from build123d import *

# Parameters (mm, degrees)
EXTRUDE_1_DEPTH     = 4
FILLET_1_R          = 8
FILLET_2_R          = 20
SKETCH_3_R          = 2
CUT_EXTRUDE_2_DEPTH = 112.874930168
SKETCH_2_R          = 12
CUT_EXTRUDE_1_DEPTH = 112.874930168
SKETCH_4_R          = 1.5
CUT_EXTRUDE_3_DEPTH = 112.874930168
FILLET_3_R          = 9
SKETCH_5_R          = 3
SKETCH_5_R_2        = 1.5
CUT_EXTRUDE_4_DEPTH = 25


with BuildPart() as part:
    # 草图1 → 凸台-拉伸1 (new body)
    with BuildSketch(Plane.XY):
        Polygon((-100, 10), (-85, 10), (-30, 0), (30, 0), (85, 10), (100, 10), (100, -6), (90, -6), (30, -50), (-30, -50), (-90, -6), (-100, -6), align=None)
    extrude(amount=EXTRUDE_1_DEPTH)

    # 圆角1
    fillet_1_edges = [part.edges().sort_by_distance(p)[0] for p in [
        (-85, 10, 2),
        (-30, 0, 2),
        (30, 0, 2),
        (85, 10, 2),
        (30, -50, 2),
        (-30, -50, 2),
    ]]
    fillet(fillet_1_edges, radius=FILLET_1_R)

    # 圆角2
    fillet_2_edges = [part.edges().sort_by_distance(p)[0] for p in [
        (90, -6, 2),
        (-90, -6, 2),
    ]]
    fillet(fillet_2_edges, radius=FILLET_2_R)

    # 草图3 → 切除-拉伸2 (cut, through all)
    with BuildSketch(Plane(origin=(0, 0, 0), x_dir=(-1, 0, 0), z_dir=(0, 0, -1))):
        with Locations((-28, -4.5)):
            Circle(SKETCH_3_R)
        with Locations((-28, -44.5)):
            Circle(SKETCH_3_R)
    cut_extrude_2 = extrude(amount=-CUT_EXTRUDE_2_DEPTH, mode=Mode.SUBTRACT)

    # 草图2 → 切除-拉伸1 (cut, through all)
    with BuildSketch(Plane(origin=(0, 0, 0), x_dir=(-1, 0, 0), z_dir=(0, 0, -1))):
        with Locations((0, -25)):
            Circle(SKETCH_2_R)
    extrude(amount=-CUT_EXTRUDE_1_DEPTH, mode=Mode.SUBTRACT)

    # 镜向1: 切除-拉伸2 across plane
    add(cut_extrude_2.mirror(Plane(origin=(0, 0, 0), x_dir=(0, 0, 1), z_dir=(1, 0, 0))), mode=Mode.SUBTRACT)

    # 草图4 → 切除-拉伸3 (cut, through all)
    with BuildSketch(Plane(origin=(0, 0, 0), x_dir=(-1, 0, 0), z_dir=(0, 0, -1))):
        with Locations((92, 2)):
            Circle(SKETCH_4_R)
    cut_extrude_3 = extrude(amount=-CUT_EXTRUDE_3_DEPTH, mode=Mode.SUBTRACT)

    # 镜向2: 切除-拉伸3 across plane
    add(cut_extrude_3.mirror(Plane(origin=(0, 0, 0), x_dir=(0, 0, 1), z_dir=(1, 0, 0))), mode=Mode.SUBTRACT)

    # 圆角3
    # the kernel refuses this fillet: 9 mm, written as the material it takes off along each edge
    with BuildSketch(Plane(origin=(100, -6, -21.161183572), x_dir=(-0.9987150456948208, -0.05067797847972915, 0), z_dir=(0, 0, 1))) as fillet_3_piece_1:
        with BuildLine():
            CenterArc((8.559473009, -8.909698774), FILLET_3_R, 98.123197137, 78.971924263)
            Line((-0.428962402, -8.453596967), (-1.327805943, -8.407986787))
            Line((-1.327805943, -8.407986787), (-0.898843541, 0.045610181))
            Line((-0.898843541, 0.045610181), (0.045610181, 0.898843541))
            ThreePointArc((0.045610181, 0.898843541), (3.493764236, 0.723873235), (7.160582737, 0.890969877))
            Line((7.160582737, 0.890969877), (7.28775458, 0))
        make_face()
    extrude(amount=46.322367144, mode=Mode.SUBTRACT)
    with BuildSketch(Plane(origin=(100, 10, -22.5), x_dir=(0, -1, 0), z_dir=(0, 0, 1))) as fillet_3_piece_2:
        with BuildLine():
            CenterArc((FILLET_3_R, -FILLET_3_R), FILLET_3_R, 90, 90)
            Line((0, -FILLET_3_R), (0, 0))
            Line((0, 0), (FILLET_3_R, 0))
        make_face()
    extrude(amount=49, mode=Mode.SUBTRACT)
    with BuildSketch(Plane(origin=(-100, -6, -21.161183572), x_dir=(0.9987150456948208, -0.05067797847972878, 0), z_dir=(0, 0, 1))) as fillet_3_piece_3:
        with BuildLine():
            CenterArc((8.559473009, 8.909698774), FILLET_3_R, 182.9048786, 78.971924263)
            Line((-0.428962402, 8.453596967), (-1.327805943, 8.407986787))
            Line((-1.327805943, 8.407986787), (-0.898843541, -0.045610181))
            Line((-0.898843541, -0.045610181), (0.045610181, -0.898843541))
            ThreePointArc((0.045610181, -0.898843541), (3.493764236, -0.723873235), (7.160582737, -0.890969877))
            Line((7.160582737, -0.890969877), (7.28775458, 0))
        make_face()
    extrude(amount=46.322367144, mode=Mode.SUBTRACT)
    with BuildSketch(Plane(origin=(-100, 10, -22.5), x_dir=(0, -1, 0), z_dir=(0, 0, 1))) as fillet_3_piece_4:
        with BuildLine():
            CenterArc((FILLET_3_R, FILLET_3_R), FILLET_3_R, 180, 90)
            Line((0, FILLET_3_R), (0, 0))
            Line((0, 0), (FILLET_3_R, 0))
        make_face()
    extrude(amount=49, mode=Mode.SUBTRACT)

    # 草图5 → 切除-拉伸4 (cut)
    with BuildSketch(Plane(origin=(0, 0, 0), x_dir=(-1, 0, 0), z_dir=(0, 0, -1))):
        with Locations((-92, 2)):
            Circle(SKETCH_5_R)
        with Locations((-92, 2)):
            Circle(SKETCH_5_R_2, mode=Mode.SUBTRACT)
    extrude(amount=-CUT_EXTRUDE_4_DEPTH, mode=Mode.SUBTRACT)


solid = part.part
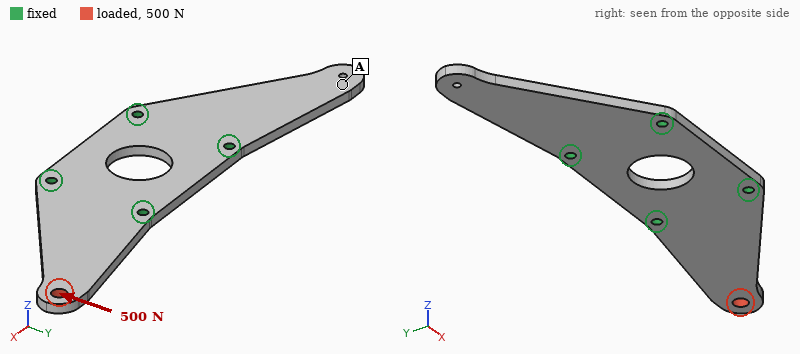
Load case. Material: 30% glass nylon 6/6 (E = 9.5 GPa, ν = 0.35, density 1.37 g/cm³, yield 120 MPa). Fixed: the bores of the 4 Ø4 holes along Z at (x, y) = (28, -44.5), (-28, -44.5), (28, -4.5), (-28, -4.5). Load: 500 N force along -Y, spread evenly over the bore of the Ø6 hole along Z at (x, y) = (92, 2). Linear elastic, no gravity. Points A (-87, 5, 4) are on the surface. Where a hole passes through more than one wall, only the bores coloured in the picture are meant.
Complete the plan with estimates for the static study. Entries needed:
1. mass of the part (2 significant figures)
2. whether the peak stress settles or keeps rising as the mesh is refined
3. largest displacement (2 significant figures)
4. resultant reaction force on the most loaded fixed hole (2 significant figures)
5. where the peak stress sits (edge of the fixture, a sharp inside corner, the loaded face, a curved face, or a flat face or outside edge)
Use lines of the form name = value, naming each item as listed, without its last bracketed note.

mass of the part = 37 g
whether the peak stress settles or keeps rising as the mesh is refined = keeps rising
largest displacement = 0.53 mm
resultant reaction force on the most loaded fixed hole = 840 N
where the peak stress sits = edge of the fixture
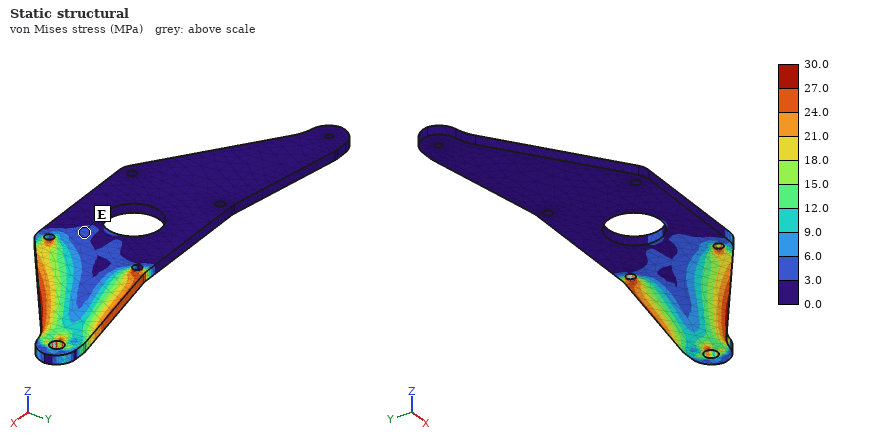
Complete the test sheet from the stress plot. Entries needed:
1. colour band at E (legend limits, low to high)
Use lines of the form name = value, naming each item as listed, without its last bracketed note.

colour band at E = 3.0 to 6.0 MPa
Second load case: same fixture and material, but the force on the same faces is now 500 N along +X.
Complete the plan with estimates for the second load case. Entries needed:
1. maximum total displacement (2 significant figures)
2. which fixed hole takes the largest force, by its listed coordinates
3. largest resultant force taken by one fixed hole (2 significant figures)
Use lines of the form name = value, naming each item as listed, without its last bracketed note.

maximum total displacement = 0.18 mm
which fixed hole takes the largest force, by its listed coordinates = (28, -4.5)
largest resultant force taken by one fixed hole = 560 N
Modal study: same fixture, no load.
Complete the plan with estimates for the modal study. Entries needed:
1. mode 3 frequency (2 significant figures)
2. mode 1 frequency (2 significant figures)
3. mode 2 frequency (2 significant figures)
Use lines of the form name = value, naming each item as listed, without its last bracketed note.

mode 3 frequency = 1900 Hz
mode 1 frequency = 440 Hz
mode 2 frequency = 450 Hz
